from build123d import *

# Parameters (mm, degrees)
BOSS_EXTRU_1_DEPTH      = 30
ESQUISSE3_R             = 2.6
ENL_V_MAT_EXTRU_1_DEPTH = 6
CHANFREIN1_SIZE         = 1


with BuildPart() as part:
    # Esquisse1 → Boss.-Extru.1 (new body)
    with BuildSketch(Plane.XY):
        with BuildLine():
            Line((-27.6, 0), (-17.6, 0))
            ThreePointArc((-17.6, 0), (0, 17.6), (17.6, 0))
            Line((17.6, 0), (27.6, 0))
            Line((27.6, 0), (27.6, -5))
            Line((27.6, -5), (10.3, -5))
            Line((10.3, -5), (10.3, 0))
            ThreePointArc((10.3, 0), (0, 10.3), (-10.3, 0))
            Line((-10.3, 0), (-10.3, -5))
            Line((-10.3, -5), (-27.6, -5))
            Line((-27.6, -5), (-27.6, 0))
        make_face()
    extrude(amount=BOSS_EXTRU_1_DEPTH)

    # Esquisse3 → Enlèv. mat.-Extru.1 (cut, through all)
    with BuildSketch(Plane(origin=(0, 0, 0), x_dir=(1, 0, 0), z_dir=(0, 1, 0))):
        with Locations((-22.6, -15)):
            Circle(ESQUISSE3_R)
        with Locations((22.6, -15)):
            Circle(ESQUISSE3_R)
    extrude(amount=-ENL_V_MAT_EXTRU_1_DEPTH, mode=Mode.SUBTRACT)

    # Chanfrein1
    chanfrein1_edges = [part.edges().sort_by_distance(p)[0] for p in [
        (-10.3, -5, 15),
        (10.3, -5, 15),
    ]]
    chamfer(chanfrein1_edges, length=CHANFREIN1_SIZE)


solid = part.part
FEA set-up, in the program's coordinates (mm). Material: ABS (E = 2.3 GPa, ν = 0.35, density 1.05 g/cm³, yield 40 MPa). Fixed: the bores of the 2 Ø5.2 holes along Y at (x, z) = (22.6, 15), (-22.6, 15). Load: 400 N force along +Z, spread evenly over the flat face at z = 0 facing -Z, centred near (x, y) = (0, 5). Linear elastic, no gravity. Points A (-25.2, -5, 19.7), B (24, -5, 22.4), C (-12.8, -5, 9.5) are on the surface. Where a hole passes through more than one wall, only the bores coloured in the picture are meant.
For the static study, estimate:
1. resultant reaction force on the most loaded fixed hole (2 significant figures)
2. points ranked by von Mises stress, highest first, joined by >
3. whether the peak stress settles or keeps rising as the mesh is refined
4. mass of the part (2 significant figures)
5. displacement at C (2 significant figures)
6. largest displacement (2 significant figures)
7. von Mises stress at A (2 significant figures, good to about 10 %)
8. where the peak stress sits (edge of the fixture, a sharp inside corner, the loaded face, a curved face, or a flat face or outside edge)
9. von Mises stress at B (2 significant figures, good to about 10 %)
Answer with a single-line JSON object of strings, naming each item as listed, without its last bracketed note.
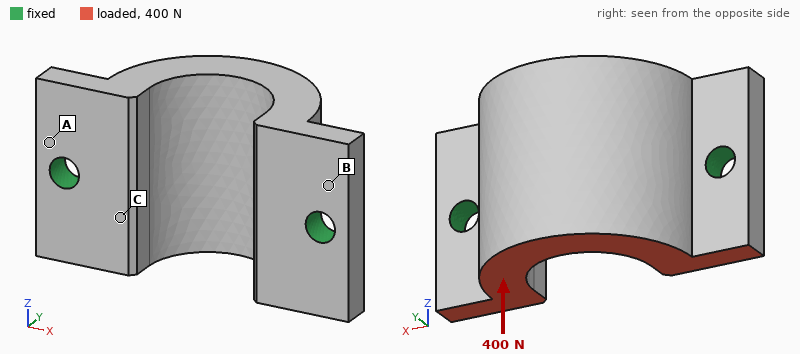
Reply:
{"resultant reaction force on the most loaded fixed hole": "200 N", "points ranked by von Mises stress, highest first, joined by >": "A > B > C", "whether the peak stress settles or keeps rising as the mesh is refined": "keeps rising", "mass of the part": "15 g", "displacement at C": "0.065 mm", "largest displacement": "0.34 mm", "von Mises stress at A": "8.7 MPa", "where the peak stress sits": "edge of the fixture", "von Mises stress at B": "5.5 MPa"}
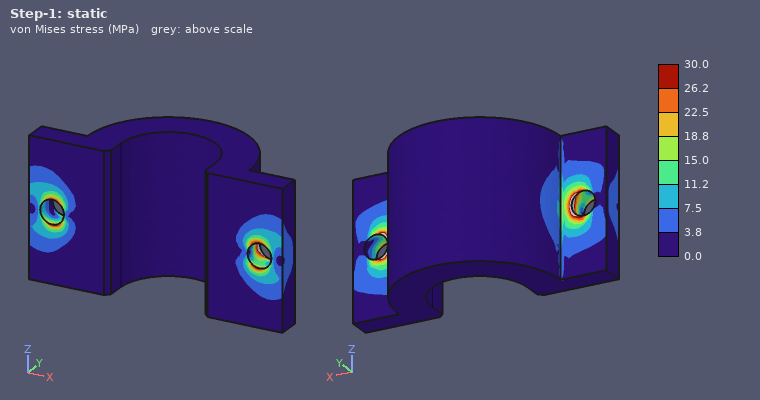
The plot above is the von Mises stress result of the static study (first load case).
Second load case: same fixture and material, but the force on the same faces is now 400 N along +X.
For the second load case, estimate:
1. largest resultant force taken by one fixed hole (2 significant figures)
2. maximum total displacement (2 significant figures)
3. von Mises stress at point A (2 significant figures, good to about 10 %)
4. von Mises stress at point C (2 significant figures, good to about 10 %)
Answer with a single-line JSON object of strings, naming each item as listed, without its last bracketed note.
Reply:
{"largest resultant force taken by one fixed hole": "230 N", "maximum total displacement": "0.11 mm", "von Mises stress at point A": "1.7 MPa", "von Mises stress at point C": "2.7 MPa"}
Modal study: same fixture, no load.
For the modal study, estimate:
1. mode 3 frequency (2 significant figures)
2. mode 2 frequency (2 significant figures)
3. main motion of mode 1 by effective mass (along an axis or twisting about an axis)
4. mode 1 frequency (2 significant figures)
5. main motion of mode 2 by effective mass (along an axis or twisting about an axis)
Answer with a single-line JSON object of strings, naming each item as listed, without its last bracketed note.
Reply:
{"mode 3 frequency": "4700 Hz", "mode 2 frequency": "4500 Hz", "main motion of mode 1 by effective mass": "along Z", "mode 1 frequency": "1600 Hz", "main motion of mode 2 by effective mass": "along Y"}
